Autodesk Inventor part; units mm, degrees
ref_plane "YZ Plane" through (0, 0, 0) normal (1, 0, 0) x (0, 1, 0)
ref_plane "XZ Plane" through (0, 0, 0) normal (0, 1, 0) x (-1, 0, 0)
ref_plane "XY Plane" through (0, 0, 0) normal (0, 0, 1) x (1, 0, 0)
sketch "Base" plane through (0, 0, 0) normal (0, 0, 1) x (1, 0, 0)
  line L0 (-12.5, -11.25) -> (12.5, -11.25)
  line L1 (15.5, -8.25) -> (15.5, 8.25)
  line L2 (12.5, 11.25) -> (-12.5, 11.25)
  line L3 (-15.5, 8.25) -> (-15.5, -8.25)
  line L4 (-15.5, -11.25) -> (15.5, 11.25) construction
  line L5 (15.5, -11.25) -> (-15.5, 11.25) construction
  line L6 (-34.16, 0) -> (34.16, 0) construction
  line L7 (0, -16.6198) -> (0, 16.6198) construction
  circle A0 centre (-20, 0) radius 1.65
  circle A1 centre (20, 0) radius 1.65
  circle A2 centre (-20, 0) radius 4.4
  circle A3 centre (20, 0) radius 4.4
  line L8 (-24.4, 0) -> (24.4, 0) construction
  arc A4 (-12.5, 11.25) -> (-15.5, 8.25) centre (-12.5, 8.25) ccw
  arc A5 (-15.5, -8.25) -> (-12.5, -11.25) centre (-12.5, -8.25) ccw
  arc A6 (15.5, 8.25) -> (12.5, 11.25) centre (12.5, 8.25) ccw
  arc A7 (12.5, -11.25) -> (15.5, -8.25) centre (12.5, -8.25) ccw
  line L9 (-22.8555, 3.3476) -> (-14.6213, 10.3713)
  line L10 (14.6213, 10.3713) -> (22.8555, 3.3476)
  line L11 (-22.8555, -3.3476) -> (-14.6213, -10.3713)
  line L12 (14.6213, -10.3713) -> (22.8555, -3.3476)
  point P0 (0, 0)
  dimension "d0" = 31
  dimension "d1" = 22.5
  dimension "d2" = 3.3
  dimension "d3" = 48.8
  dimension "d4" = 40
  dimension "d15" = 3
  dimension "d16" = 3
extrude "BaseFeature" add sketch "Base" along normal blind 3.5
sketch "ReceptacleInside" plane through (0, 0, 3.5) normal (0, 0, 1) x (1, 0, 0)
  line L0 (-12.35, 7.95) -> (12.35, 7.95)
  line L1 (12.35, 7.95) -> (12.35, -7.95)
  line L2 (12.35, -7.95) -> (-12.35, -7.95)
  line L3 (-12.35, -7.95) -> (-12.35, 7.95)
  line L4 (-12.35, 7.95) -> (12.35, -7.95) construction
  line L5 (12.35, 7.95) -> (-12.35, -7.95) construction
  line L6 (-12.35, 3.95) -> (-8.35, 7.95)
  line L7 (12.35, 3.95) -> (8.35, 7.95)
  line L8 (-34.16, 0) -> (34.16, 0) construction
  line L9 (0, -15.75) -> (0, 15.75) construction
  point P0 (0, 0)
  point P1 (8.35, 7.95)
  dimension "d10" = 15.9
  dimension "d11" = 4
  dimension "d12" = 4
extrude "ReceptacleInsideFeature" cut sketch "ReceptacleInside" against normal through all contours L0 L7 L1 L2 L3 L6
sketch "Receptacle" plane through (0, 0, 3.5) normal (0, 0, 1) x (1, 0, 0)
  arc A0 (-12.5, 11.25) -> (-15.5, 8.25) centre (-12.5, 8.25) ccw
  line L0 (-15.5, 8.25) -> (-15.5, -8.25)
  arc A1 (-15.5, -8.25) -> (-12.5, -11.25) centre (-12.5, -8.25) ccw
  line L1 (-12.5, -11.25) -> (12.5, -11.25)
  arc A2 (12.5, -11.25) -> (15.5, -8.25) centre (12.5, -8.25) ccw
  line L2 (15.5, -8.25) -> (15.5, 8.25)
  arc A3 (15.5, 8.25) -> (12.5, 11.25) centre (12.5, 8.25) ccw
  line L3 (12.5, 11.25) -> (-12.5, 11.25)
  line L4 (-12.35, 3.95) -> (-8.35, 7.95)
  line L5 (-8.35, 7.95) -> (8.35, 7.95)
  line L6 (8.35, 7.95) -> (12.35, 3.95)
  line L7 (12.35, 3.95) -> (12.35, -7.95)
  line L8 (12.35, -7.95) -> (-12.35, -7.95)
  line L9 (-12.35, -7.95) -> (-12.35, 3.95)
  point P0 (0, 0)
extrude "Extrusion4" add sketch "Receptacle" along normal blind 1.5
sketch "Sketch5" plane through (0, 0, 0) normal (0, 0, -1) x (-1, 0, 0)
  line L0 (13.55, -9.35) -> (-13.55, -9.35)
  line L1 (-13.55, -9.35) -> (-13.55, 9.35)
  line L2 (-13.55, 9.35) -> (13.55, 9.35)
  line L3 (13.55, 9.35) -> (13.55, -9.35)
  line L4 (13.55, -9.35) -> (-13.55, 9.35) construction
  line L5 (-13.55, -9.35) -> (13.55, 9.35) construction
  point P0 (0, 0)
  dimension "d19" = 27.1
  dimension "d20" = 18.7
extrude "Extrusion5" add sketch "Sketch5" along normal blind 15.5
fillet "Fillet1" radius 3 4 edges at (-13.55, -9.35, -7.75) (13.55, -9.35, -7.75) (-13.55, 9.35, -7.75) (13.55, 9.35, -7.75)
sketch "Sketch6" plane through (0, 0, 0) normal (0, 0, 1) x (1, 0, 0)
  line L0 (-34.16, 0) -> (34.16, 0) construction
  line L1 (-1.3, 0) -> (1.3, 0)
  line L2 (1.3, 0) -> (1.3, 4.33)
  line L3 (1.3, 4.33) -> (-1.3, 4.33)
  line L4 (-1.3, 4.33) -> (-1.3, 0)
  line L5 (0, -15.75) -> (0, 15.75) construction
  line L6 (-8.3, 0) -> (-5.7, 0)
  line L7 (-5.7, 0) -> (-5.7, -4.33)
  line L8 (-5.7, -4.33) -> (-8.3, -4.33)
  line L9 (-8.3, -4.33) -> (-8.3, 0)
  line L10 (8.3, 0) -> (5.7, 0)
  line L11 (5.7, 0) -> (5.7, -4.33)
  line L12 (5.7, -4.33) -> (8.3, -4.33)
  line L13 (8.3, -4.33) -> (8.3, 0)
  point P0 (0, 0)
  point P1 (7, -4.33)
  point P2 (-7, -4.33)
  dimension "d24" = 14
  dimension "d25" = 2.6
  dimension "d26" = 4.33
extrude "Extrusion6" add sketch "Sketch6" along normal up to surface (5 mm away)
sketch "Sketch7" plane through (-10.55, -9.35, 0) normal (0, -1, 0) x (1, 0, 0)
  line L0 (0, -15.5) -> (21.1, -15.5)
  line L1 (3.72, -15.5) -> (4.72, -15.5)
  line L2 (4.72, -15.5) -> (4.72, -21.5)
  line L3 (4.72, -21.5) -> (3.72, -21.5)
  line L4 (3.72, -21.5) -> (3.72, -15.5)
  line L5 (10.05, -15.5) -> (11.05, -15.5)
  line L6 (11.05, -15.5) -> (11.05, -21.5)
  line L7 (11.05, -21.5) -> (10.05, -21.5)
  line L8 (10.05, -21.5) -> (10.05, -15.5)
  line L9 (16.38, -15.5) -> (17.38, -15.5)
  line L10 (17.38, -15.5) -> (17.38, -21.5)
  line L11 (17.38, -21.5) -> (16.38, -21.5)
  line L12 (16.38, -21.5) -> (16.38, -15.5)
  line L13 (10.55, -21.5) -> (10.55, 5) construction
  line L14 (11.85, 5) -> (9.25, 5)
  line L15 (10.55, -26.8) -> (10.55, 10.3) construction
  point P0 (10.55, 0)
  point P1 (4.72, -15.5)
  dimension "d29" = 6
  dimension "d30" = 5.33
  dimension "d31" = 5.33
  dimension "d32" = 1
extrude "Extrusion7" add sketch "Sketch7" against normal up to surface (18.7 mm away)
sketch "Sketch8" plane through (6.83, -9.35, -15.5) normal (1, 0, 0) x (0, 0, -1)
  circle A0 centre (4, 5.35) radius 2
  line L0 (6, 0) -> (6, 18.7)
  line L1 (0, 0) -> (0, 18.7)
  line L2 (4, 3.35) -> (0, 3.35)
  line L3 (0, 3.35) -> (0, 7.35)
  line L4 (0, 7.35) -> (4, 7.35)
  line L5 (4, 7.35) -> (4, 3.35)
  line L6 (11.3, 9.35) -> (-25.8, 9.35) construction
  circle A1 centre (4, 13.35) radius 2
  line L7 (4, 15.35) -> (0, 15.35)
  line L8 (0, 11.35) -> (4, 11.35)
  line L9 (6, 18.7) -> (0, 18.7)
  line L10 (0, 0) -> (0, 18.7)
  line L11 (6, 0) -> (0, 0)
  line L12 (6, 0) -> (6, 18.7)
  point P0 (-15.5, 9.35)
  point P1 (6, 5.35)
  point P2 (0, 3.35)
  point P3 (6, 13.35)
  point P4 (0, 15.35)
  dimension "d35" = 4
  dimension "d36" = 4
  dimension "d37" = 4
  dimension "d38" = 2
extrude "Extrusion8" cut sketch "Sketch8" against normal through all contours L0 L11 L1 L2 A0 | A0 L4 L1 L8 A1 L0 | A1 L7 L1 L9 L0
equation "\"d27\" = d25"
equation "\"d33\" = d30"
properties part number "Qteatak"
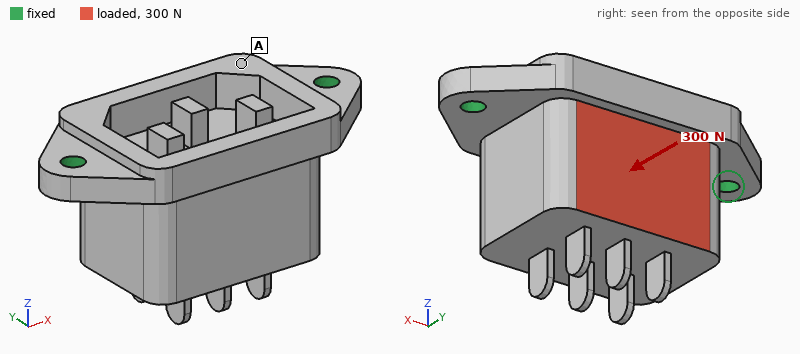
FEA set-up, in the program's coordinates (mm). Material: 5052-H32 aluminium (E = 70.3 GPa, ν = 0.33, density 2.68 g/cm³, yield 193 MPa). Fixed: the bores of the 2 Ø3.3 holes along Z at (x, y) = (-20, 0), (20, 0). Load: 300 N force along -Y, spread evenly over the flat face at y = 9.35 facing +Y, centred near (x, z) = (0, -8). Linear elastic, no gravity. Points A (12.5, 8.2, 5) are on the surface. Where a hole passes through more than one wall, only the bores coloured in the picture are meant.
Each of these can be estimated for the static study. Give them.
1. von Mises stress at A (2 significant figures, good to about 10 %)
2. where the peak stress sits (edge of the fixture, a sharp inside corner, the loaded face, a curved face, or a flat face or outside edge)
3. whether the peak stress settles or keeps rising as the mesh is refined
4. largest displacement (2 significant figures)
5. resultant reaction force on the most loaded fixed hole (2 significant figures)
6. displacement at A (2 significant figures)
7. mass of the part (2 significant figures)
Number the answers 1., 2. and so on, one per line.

1. 10 MPa
2. edge of the fixture
3. keeps rising
4. 37 µm
5. 150 N
6. 12 µm
7. 28 g
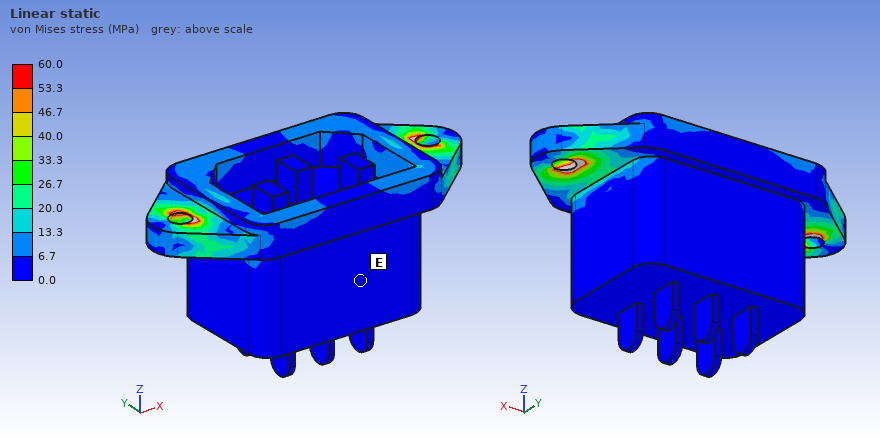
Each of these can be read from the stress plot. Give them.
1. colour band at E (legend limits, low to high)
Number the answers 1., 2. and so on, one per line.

1. 0.0 to 6.7 MPa
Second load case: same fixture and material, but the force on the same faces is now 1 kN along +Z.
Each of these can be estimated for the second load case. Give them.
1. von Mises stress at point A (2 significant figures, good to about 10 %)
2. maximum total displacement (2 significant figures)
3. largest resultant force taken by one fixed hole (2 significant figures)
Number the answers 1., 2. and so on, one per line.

1. 44 MPa
2. 0.12 mm
3. 590 N
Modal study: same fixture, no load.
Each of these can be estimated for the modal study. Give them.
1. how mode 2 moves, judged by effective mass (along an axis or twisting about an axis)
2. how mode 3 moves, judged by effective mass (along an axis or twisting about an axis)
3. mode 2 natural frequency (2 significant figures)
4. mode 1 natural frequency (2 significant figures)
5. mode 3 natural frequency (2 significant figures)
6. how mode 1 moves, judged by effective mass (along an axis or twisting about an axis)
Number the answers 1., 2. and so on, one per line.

1. along Z
2. along X
3. 9700 Hz
4. 3700 Hz
5. 12 kHz
6. along Y
